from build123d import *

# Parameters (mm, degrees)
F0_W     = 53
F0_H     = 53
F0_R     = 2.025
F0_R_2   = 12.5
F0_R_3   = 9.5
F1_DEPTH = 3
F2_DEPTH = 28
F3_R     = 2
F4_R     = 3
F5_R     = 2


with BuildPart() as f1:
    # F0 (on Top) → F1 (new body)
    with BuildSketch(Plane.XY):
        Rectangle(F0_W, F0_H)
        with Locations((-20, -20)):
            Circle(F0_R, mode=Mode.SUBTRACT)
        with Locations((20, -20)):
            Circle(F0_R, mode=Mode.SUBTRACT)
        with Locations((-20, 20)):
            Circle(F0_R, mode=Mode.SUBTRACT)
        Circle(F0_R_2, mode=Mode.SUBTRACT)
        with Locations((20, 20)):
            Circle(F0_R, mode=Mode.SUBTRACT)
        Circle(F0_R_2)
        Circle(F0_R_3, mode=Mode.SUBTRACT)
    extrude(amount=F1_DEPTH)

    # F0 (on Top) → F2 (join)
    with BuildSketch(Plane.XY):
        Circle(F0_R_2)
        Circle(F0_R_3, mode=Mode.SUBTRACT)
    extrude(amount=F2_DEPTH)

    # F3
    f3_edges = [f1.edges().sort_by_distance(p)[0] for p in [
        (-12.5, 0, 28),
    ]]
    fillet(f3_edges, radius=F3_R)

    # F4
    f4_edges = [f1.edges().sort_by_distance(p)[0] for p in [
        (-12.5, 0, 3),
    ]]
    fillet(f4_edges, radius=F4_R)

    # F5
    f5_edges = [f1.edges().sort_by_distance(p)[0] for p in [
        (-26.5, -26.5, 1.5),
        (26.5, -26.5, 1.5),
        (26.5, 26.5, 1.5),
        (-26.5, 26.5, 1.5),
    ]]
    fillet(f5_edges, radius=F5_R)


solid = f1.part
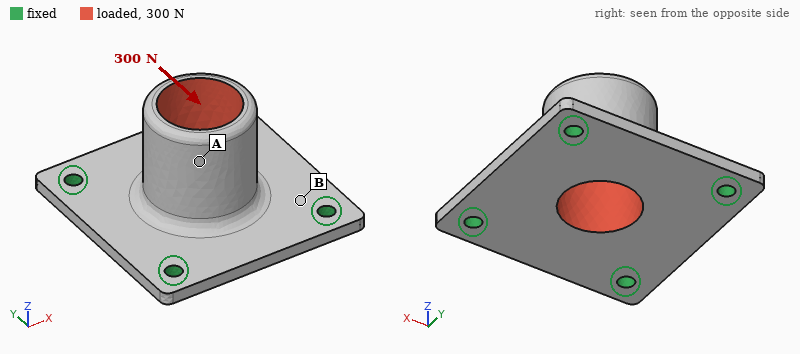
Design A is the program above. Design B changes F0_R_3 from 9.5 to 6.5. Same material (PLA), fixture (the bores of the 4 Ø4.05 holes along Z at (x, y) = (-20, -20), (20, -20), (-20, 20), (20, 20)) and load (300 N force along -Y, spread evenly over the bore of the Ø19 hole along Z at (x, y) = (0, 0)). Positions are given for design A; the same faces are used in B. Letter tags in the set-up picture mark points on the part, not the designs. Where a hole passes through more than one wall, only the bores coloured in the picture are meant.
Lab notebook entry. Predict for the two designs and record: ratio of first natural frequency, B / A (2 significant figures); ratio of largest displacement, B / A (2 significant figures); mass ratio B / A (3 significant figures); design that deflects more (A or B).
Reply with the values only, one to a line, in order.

0.85
0.87
1.33
A
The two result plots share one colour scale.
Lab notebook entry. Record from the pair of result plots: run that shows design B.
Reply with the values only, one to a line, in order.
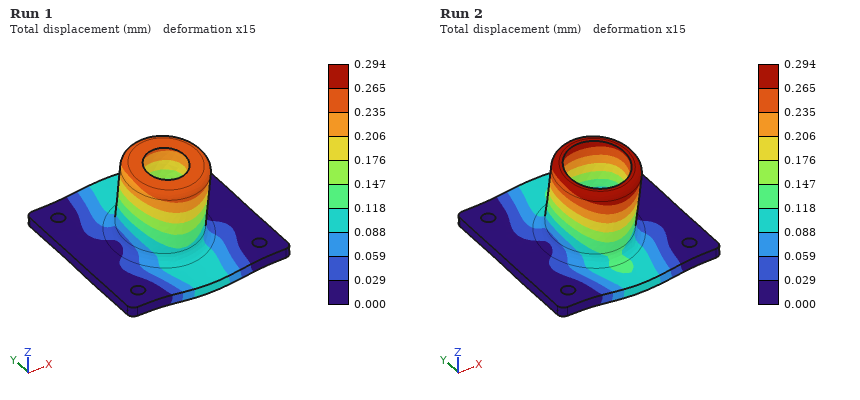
Run 1
